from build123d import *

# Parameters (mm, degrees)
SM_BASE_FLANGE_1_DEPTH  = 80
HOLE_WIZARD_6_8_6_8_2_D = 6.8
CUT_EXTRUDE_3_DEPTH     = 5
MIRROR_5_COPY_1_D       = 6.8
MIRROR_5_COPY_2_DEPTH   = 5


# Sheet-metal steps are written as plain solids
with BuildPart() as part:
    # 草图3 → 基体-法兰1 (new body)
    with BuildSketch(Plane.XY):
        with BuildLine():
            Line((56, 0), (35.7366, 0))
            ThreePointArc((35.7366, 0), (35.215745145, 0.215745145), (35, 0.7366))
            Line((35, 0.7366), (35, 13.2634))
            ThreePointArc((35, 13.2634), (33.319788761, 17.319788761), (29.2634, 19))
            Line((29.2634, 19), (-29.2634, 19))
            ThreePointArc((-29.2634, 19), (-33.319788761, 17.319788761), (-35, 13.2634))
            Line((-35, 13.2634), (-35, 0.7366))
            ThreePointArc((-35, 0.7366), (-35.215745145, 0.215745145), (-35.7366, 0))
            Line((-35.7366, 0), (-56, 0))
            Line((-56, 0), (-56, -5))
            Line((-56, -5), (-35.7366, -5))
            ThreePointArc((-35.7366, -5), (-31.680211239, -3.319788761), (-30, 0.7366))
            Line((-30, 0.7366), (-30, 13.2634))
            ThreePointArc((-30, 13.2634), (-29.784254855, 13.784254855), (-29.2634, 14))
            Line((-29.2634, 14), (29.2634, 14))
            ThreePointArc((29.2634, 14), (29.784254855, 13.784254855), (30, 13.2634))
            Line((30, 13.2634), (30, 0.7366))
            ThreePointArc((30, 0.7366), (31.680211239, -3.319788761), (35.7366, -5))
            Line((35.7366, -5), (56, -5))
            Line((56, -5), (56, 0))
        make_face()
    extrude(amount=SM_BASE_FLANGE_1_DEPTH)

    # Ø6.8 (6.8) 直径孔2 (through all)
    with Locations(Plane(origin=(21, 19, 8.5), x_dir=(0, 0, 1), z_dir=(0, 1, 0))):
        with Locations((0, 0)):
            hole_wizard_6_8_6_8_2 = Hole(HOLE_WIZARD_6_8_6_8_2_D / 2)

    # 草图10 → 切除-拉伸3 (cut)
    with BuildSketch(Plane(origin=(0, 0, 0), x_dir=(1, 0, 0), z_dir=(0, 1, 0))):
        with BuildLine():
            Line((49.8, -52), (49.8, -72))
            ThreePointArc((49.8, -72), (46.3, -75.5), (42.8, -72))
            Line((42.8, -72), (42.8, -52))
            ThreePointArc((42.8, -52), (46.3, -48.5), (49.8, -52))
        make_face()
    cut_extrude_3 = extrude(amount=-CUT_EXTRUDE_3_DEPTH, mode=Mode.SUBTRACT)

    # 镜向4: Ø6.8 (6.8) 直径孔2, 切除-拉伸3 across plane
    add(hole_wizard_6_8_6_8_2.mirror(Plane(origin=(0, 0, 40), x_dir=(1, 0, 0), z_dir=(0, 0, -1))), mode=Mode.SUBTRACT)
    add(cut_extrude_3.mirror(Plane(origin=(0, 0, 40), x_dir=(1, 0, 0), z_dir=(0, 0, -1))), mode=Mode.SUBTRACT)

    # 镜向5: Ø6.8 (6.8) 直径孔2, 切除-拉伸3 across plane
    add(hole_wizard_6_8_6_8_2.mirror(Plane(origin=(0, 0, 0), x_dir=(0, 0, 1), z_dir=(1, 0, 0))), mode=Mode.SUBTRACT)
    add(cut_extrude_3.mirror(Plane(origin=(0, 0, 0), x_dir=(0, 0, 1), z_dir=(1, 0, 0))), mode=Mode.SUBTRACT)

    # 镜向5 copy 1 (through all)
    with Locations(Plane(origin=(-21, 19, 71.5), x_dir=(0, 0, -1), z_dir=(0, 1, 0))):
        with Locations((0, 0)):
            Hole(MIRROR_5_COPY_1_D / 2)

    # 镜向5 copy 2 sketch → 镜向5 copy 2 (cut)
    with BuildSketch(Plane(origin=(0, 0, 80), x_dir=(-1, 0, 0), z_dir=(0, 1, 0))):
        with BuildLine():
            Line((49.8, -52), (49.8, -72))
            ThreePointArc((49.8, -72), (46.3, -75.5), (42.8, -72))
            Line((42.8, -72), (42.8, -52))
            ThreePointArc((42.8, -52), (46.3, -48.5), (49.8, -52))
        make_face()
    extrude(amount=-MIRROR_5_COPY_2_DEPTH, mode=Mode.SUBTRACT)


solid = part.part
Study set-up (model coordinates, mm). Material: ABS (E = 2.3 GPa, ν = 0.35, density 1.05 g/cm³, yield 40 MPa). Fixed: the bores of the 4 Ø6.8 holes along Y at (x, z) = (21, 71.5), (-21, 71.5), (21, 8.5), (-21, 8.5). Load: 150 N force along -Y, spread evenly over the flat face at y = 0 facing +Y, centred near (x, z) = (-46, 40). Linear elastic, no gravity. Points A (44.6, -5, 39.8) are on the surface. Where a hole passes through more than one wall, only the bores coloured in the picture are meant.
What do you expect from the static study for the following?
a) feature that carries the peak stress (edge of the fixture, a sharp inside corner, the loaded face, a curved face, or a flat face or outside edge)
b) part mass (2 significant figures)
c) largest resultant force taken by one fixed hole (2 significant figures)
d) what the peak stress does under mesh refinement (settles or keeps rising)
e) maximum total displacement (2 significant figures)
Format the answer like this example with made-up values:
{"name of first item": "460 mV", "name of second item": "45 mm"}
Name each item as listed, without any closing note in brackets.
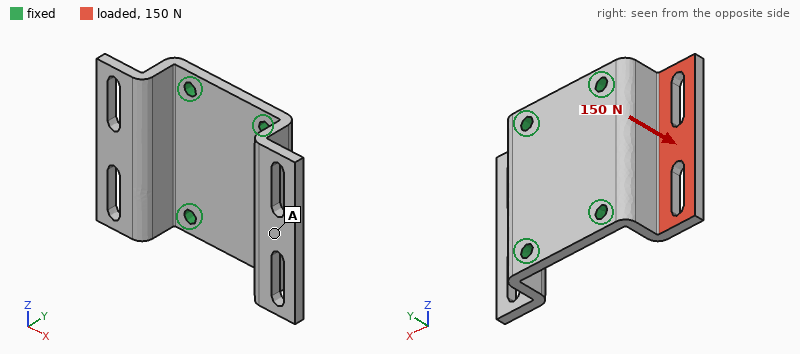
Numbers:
{"feature that carries the peak stress": "edge of the fixture", "part mass": "56 g", "largest resultant force taken by one fixed hole": "94 N", "what the peak stress does under mesh refinement": "keeps rising", "maximum total displacement": "1.3 mm"}
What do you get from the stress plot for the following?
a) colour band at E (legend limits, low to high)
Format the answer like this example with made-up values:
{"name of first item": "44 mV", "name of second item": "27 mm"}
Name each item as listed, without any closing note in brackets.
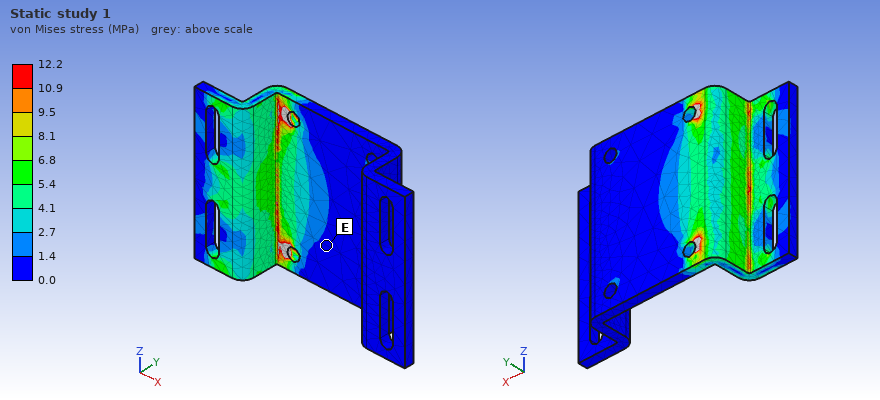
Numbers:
{"colour band at E": "0.0 to 1.4 MPa"}
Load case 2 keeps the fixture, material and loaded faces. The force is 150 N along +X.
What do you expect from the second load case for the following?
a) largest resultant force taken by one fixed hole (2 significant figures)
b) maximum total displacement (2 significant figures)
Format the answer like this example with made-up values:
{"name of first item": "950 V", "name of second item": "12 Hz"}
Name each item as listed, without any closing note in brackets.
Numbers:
{"largest resultant force taken by one fixed hole": "55 N", "maximum total displacement": "0.72 mm"}
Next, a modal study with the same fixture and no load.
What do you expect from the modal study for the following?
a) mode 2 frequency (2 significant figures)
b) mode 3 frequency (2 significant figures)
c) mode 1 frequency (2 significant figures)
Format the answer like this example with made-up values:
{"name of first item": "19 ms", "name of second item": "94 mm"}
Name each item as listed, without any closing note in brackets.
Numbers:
{"mode 2 frequency": "650 Hz", "mode 3 frequency": "1100 Hz", "mode 1 frequency": "630 Hz"}
